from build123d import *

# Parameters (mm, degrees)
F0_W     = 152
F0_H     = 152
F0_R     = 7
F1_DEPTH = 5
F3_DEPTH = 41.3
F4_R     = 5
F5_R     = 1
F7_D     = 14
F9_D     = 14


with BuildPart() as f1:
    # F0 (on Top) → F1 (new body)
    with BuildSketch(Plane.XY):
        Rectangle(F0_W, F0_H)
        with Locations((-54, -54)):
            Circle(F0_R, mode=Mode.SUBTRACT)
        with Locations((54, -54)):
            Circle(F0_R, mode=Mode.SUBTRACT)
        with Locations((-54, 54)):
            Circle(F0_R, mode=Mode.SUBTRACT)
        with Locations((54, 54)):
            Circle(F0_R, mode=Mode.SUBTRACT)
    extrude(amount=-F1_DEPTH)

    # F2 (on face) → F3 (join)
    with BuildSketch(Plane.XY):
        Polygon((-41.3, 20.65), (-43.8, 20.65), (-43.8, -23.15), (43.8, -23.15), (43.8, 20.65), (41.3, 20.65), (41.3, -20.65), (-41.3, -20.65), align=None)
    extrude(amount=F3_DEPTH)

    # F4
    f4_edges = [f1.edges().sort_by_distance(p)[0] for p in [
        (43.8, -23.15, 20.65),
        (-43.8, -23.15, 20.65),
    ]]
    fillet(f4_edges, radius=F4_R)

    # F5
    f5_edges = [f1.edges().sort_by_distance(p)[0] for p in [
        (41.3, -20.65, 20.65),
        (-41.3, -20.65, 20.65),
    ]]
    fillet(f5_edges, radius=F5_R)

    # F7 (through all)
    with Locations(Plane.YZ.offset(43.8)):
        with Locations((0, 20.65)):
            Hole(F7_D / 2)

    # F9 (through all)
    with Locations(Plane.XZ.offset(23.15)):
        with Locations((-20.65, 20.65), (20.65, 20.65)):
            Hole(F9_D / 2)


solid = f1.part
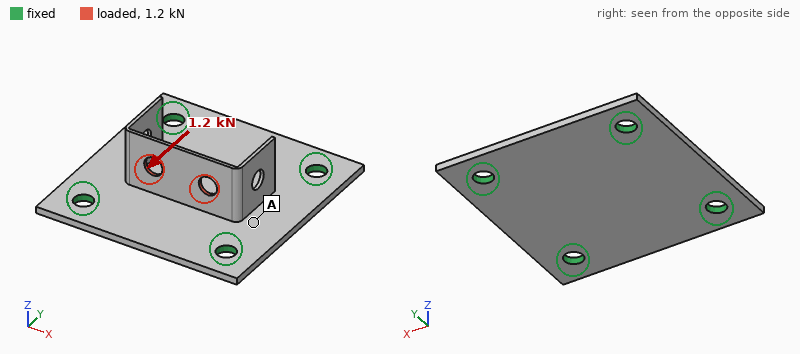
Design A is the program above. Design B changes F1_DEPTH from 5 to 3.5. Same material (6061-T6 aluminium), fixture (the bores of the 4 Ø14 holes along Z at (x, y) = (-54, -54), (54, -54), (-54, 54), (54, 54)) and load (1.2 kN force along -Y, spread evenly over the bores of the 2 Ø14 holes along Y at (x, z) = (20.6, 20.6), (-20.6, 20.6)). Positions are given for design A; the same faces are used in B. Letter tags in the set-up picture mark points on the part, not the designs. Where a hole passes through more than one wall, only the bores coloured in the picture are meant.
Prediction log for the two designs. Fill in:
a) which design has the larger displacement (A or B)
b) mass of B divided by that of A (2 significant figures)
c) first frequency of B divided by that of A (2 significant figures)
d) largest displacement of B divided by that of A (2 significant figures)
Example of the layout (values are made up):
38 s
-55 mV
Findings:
B
0.74
0.82
1.1
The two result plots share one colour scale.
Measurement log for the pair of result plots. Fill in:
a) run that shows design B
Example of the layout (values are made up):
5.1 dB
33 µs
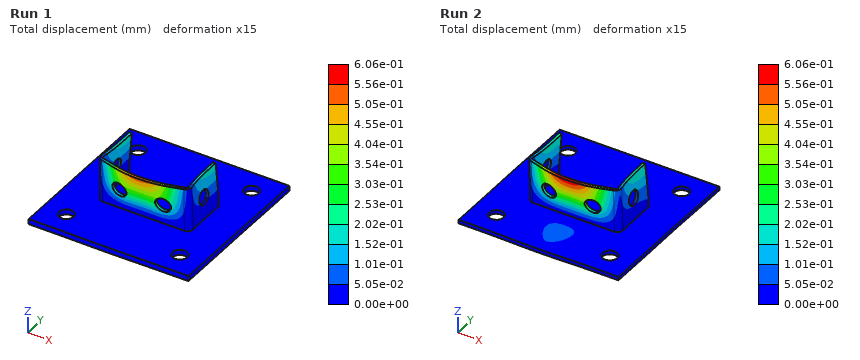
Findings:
Run 2
